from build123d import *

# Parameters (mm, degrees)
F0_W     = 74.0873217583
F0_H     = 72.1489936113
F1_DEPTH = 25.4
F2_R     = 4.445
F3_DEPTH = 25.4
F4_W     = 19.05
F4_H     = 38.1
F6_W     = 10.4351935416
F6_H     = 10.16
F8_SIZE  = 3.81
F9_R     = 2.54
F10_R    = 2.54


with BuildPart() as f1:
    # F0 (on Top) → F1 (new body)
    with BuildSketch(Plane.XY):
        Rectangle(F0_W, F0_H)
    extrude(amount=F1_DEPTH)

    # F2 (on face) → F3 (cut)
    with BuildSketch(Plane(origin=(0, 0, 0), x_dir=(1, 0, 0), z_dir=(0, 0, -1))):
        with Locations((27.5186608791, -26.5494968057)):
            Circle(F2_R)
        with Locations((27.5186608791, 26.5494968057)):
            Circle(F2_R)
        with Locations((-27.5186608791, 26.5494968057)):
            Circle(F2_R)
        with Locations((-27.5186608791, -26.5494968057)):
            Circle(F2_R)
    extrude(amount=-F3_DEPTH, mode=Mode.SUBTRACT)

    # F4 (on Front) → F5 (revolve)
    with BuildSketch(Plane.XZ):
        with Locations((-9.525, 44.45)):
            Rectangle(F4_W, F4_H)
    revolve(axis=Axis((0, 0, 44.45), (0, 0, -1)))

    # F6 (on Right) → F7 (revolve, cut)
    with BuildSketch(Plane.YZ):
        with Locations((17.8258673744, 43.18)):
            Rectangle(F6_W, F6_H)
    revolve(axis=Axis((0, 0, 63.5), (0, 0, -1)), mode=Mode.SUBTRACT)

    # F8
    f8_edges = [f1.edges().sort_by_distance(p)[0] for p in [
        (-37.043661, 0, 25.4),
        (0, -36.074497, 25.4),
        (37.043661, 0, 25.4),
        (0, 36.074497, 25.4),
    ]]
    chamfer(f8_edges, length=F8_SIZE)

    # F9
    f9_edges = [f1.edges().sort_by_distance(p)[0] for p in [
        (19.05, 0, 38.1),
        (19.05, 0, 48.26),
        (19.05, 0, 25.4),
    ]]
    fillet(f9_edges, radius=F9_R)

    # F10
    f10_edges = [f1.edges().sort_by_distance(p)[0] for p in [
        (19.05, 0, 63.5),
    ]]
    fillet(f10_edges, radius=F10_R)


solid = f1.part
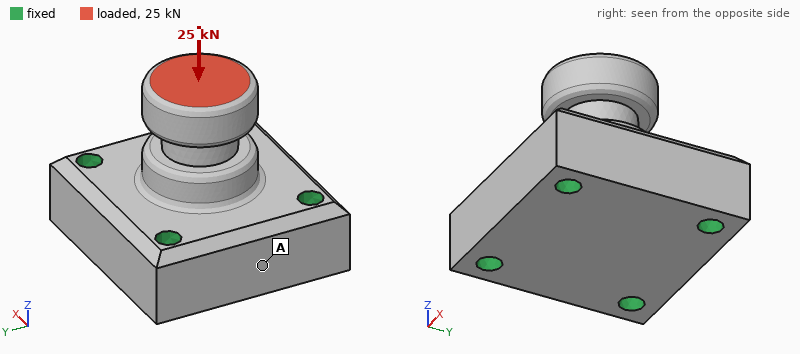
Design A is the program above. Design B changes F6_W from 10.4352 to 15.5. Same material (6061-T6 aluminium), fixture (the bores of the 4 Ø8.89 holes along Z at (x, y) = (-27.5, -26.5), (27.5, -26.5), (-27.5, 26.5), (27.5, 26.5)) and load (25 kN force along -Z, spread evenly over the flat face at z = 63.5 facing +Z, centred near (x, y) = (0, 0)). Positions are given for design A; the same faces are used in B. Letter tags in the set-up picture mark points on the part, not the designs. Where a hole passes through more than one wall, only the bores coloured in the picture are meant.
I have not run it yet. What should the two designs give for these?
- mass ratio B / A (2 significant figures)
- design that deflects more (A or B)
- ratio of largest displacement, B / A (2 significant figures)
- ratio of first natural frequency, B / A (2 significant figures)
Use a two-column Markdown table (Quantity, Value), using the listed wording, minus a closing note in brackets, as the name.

| Quantity | Value |
|---|---|
| mass ratio B / A | 0.99 |
| design that deflects more | B |
| ratio of largest displacement, B / A | 1.3 |
| ratio of first natural frequency, B / A | 0.79 |
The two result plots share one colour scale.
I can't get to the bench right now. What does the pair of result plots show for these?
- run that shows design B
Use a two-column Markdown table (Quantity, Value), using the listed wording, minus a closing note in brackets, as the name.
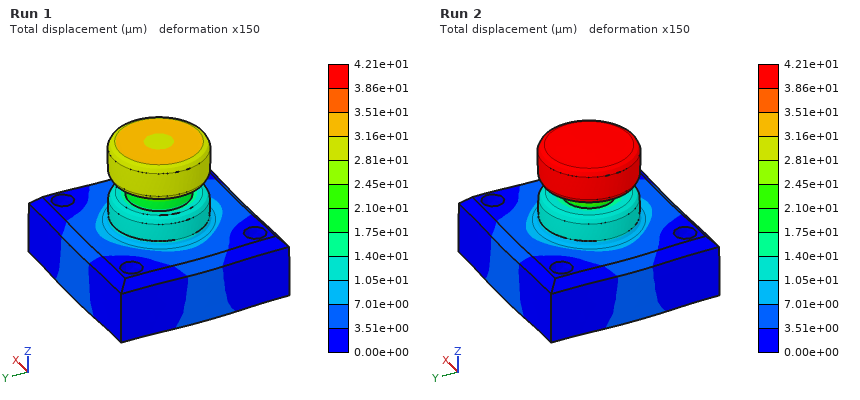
| Quantity | Value |
|---|---|
| run that shows design B | Run 2 |
